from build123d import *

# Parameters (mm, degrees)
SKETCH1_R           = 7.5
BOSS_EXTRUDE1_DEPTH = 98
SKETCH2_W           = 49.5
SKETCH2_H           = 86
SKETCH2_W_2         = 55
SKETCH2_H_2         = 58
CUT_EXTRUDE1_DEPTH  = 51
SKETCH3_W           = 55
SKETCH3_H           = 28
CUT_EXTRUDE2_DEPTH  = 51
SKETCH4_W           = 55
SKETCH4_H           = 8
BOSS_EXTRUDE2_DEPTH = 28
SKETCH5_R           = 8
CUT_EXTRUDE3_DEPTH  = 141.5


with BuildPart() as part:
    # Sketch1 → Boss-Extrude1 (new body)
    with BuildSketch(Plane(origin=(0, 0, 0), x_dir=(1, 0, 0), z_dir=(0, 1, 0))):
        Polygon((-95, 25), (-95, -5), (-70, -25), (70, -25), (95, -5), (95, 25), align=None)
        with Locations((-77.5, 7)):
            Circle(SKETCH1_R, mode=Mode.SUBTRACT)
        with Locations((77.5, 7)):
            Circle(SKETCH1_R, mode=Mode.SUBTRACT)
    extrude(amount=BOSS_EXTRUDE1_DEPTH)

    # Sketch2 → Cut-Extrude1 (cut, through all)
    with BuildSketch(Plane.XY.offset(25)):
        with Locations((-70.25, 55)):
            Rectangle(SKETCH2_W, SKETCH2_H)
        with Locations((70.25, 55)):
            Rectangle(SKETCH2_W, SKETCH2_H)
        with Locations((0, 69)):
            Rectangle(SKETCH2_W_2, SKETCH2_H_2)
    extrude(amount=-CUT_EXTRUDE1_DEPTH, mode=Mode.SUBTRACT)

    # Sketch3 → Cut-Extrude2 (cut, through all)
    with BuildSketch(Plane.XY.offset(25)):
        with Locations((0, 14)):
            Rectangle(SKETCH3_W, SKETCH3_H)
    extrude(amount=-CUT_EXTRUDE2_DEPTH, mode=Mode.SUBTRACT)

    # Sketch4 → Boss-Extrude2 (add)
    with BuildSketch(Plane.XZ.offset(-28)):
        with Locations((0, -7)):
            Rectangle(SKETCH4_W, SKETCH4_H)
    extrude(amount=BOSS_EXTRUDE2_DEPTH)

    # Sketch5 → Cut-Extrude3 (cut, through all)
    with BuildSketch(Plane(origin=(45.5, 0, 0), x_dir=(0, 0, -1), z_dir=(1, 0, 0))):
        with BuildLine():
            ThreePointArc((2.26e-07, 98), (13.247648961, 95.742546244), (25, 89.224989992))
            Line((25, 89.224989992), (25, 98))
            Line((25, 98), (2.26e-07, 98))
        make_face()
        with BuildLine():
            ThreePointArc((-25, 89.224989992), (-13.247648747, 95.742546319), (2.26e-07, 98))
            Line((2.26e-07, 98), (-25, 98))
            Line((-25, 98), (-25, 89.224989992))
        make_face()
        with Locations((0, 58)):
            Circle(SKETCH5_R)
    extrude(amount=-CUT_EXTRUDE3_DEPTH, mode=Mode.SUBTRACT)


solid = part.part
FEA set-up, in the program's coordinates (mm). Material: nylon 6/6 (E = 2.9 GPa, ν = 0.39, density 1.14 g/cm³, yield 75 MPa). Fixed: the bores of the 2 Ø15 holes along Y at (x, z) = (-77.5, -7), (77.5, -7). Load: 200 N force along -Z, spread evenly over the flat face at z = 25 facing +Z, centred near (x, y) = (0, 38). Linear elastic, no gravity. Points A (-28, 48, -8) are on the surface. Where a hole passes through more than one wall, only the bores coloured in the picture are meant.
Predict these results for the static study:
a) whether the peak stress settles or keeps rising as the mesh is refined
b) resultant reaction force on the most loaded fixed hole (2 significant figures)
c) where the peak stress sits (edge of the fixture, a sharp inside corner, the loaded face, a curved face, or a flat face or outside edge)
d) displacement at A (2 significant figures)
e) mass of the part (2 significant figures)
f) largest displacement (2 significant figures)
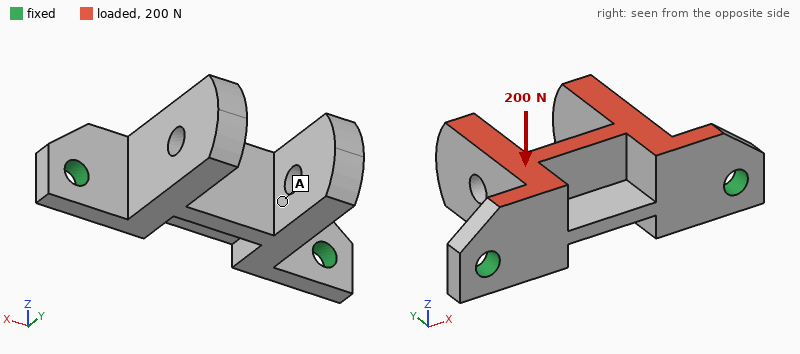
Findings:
keeps rising
100 N
edge of the fixture
0.16 mm
290 g
0.33 mm
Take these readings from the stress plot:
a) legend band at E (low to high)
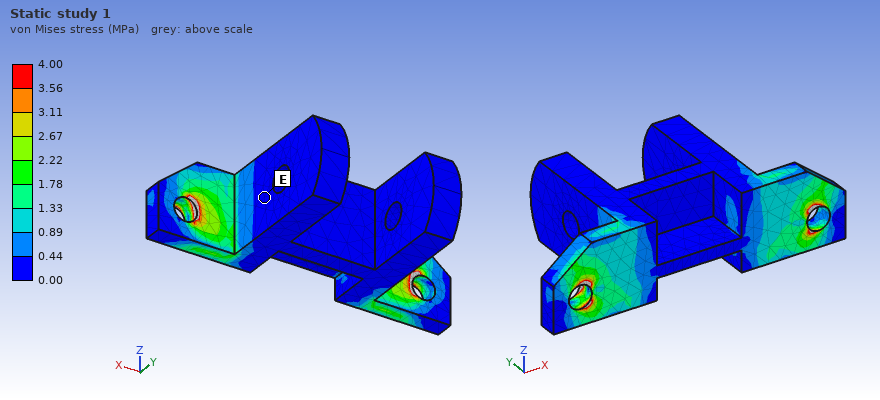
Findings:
0.00 to 0.44 MPa
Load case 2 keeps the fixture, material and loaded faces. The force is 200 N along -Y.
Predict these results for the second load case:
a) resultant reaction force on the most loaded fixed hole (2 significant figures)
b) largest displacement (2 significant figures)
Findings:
120 N
0.27 mm
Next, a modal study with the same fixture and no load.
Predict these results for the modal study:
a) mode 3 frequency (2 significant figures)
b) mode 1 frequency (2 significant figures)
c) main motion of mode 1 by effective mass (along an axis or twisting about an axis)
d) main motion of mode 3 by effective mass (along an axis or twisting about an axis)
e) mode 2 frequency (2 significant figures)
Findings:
700 Hz
290 Hz
along Z
along X
590 Hz
